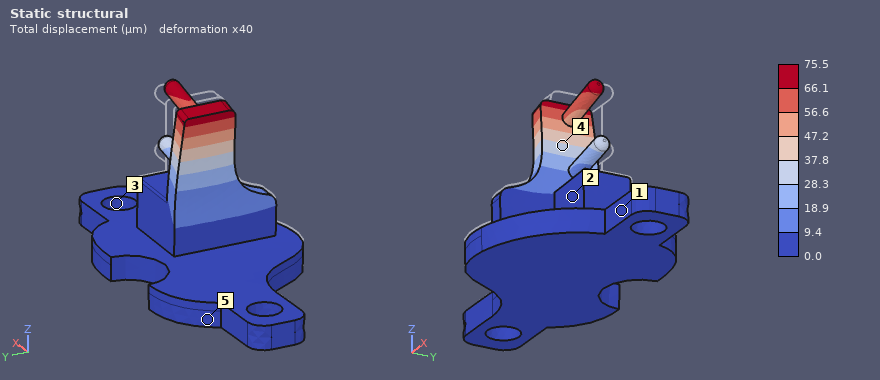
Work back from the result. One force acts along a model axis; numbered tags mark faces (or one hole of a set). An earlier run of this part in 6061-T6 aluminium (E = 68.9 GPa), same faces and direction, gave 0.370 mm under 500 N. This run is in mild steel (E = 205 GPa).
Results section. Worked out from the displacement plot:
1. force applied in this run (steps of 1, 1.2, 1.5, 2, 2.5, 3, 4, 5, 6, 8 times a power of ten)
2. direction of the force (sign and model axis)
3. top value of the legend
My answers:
300 N
-X
75.5 µm
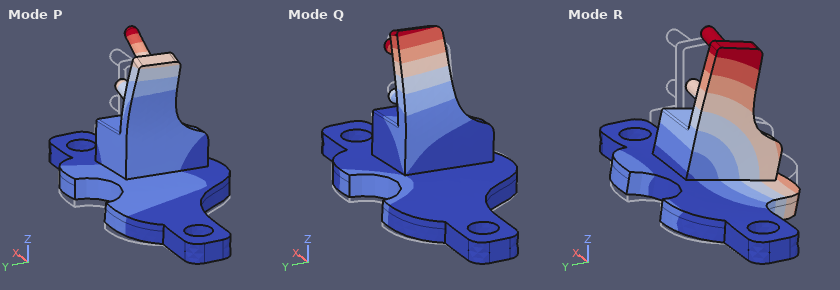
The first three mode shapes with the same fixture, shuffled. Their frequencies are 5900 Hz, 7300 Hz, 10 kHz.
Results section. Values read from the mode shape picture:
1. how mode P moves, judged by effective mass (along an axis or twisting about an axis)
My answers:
along Z
